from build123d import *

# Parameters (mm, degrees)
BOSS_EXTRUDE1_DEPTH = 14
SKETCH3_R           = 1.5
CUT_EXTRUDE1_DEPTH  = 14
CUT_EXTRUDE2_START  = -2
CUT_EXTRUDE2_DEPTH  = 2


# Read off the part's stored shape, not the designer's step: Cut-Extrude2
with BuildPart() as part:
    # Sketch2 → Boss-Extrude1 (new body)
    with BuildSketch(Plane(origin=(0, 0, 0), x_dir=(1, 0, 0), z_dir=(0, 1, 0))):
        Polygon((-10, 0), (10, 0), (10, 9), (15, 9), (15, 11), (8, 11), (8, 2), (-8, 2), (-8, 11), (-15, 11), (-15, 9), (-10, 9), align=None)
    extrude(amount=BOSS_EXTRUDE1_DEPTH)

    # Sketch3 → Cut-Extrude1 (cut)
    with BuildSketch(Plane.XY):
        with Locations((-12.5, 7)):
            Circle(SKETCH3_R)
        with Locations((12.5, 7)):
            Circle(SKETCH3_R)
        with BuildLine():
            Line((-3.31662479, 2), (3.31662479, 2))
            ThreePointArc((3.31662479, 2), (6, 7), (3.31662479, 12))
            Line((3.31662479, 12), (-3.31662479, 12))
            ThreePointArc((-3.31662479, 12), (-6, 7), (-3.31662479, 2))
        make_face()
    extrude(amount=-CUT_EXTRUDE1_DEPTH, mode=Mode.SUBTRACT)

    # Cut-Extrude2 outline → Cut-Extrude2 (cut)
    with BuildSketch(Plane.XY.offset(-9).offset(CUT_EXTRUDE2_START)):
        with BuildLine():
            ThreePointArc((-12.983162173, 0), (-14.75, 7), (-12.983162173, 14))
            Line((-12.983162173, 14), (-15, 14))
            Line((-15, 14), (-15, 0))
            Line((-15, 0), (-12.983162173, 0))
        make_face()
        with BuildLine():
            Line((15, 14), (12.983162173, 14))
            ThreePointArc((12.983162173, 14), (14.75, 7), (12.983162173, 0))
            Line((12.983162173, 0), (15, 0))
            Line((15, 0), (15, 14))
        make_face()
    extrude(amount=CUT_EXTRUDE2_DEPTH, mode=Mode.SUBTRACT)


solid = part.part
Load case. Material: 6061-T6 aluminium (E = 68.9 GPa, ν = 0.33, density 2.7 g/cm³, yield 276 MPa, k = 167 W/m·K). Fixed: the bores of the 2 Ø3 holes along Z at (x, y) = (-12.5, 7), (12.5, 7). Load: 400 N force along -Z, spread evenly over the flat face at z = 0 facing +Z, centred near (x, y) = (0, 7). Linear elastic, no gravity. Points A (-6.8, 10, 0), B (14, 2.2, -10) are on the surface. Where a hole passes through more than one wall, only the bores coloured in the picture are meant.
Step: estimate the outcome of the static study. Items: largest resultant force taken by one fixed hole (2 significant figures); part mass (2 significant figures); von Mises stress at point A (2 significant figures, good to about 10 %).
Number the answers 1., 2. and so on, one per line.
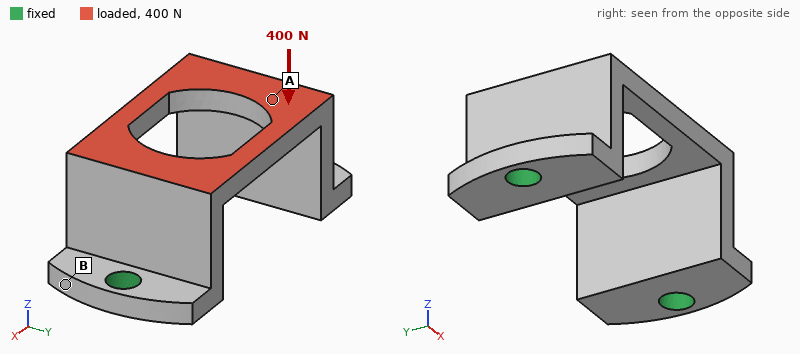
1. 210 N
2. 2.9 g
3. 17 MPa
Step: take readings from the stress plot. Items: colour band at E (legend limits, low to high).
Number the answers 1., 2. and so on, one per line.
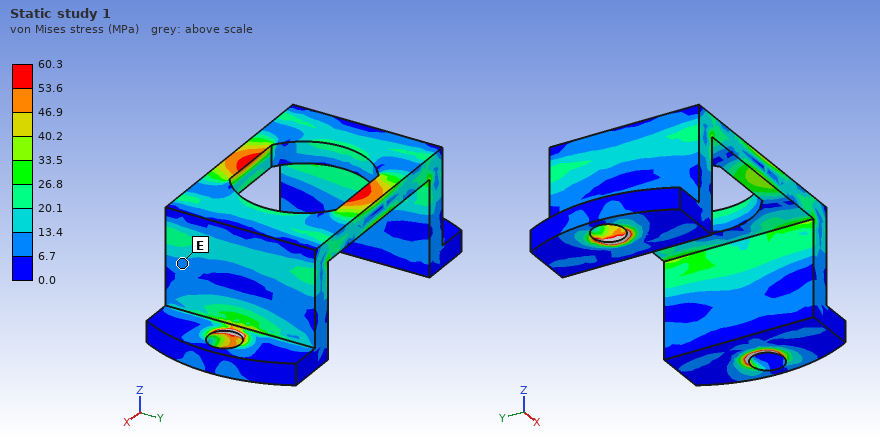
1. 6.7 to 13.4 MPa
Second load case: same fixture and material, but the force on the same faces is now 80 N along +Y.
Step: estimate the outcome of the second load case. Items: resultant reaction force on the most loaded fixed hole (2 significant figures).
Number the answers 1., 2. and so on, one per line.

1. 40 N
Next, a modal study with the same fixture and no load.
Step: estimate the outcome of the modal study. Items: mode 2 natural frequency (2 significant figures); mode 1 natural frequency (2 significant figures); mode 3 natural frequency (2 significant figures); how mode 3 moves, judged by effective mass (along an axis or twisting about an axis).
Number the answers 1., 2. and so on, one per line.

1. 11 kHz
2. 11 kHz
3. 14 kHz
4. twisting about Z
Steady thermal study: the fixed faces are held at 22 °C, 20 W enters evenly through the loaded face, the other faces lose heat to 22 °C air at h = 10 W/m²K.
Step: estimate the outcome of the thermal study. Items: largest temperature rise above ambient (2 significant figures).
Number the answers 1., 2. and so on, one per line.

1. 35 K
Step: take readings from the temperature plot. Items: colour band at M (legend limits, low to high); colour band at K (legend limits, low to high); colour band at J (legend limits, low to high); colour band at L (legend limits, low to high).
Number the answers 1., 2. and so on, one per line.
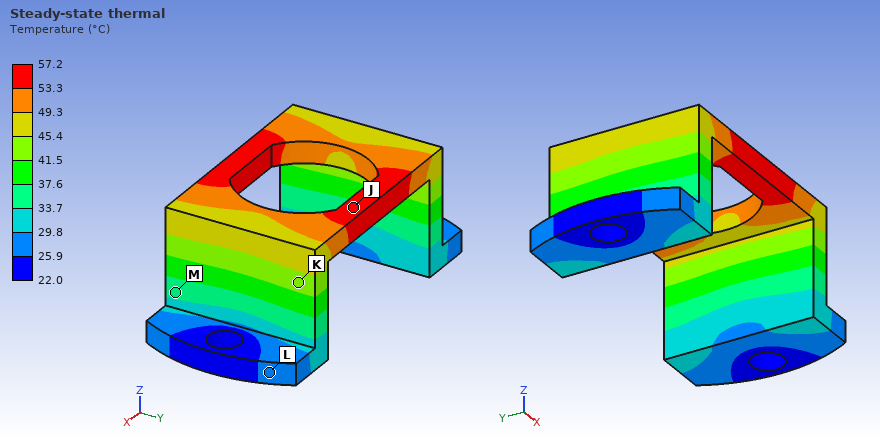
1. 33.7 to 37.6 °C
2. 41.5 to 45.4 °C
3. 53.3 to 57.2 °C
4. 25.9 to 29.8 °C
